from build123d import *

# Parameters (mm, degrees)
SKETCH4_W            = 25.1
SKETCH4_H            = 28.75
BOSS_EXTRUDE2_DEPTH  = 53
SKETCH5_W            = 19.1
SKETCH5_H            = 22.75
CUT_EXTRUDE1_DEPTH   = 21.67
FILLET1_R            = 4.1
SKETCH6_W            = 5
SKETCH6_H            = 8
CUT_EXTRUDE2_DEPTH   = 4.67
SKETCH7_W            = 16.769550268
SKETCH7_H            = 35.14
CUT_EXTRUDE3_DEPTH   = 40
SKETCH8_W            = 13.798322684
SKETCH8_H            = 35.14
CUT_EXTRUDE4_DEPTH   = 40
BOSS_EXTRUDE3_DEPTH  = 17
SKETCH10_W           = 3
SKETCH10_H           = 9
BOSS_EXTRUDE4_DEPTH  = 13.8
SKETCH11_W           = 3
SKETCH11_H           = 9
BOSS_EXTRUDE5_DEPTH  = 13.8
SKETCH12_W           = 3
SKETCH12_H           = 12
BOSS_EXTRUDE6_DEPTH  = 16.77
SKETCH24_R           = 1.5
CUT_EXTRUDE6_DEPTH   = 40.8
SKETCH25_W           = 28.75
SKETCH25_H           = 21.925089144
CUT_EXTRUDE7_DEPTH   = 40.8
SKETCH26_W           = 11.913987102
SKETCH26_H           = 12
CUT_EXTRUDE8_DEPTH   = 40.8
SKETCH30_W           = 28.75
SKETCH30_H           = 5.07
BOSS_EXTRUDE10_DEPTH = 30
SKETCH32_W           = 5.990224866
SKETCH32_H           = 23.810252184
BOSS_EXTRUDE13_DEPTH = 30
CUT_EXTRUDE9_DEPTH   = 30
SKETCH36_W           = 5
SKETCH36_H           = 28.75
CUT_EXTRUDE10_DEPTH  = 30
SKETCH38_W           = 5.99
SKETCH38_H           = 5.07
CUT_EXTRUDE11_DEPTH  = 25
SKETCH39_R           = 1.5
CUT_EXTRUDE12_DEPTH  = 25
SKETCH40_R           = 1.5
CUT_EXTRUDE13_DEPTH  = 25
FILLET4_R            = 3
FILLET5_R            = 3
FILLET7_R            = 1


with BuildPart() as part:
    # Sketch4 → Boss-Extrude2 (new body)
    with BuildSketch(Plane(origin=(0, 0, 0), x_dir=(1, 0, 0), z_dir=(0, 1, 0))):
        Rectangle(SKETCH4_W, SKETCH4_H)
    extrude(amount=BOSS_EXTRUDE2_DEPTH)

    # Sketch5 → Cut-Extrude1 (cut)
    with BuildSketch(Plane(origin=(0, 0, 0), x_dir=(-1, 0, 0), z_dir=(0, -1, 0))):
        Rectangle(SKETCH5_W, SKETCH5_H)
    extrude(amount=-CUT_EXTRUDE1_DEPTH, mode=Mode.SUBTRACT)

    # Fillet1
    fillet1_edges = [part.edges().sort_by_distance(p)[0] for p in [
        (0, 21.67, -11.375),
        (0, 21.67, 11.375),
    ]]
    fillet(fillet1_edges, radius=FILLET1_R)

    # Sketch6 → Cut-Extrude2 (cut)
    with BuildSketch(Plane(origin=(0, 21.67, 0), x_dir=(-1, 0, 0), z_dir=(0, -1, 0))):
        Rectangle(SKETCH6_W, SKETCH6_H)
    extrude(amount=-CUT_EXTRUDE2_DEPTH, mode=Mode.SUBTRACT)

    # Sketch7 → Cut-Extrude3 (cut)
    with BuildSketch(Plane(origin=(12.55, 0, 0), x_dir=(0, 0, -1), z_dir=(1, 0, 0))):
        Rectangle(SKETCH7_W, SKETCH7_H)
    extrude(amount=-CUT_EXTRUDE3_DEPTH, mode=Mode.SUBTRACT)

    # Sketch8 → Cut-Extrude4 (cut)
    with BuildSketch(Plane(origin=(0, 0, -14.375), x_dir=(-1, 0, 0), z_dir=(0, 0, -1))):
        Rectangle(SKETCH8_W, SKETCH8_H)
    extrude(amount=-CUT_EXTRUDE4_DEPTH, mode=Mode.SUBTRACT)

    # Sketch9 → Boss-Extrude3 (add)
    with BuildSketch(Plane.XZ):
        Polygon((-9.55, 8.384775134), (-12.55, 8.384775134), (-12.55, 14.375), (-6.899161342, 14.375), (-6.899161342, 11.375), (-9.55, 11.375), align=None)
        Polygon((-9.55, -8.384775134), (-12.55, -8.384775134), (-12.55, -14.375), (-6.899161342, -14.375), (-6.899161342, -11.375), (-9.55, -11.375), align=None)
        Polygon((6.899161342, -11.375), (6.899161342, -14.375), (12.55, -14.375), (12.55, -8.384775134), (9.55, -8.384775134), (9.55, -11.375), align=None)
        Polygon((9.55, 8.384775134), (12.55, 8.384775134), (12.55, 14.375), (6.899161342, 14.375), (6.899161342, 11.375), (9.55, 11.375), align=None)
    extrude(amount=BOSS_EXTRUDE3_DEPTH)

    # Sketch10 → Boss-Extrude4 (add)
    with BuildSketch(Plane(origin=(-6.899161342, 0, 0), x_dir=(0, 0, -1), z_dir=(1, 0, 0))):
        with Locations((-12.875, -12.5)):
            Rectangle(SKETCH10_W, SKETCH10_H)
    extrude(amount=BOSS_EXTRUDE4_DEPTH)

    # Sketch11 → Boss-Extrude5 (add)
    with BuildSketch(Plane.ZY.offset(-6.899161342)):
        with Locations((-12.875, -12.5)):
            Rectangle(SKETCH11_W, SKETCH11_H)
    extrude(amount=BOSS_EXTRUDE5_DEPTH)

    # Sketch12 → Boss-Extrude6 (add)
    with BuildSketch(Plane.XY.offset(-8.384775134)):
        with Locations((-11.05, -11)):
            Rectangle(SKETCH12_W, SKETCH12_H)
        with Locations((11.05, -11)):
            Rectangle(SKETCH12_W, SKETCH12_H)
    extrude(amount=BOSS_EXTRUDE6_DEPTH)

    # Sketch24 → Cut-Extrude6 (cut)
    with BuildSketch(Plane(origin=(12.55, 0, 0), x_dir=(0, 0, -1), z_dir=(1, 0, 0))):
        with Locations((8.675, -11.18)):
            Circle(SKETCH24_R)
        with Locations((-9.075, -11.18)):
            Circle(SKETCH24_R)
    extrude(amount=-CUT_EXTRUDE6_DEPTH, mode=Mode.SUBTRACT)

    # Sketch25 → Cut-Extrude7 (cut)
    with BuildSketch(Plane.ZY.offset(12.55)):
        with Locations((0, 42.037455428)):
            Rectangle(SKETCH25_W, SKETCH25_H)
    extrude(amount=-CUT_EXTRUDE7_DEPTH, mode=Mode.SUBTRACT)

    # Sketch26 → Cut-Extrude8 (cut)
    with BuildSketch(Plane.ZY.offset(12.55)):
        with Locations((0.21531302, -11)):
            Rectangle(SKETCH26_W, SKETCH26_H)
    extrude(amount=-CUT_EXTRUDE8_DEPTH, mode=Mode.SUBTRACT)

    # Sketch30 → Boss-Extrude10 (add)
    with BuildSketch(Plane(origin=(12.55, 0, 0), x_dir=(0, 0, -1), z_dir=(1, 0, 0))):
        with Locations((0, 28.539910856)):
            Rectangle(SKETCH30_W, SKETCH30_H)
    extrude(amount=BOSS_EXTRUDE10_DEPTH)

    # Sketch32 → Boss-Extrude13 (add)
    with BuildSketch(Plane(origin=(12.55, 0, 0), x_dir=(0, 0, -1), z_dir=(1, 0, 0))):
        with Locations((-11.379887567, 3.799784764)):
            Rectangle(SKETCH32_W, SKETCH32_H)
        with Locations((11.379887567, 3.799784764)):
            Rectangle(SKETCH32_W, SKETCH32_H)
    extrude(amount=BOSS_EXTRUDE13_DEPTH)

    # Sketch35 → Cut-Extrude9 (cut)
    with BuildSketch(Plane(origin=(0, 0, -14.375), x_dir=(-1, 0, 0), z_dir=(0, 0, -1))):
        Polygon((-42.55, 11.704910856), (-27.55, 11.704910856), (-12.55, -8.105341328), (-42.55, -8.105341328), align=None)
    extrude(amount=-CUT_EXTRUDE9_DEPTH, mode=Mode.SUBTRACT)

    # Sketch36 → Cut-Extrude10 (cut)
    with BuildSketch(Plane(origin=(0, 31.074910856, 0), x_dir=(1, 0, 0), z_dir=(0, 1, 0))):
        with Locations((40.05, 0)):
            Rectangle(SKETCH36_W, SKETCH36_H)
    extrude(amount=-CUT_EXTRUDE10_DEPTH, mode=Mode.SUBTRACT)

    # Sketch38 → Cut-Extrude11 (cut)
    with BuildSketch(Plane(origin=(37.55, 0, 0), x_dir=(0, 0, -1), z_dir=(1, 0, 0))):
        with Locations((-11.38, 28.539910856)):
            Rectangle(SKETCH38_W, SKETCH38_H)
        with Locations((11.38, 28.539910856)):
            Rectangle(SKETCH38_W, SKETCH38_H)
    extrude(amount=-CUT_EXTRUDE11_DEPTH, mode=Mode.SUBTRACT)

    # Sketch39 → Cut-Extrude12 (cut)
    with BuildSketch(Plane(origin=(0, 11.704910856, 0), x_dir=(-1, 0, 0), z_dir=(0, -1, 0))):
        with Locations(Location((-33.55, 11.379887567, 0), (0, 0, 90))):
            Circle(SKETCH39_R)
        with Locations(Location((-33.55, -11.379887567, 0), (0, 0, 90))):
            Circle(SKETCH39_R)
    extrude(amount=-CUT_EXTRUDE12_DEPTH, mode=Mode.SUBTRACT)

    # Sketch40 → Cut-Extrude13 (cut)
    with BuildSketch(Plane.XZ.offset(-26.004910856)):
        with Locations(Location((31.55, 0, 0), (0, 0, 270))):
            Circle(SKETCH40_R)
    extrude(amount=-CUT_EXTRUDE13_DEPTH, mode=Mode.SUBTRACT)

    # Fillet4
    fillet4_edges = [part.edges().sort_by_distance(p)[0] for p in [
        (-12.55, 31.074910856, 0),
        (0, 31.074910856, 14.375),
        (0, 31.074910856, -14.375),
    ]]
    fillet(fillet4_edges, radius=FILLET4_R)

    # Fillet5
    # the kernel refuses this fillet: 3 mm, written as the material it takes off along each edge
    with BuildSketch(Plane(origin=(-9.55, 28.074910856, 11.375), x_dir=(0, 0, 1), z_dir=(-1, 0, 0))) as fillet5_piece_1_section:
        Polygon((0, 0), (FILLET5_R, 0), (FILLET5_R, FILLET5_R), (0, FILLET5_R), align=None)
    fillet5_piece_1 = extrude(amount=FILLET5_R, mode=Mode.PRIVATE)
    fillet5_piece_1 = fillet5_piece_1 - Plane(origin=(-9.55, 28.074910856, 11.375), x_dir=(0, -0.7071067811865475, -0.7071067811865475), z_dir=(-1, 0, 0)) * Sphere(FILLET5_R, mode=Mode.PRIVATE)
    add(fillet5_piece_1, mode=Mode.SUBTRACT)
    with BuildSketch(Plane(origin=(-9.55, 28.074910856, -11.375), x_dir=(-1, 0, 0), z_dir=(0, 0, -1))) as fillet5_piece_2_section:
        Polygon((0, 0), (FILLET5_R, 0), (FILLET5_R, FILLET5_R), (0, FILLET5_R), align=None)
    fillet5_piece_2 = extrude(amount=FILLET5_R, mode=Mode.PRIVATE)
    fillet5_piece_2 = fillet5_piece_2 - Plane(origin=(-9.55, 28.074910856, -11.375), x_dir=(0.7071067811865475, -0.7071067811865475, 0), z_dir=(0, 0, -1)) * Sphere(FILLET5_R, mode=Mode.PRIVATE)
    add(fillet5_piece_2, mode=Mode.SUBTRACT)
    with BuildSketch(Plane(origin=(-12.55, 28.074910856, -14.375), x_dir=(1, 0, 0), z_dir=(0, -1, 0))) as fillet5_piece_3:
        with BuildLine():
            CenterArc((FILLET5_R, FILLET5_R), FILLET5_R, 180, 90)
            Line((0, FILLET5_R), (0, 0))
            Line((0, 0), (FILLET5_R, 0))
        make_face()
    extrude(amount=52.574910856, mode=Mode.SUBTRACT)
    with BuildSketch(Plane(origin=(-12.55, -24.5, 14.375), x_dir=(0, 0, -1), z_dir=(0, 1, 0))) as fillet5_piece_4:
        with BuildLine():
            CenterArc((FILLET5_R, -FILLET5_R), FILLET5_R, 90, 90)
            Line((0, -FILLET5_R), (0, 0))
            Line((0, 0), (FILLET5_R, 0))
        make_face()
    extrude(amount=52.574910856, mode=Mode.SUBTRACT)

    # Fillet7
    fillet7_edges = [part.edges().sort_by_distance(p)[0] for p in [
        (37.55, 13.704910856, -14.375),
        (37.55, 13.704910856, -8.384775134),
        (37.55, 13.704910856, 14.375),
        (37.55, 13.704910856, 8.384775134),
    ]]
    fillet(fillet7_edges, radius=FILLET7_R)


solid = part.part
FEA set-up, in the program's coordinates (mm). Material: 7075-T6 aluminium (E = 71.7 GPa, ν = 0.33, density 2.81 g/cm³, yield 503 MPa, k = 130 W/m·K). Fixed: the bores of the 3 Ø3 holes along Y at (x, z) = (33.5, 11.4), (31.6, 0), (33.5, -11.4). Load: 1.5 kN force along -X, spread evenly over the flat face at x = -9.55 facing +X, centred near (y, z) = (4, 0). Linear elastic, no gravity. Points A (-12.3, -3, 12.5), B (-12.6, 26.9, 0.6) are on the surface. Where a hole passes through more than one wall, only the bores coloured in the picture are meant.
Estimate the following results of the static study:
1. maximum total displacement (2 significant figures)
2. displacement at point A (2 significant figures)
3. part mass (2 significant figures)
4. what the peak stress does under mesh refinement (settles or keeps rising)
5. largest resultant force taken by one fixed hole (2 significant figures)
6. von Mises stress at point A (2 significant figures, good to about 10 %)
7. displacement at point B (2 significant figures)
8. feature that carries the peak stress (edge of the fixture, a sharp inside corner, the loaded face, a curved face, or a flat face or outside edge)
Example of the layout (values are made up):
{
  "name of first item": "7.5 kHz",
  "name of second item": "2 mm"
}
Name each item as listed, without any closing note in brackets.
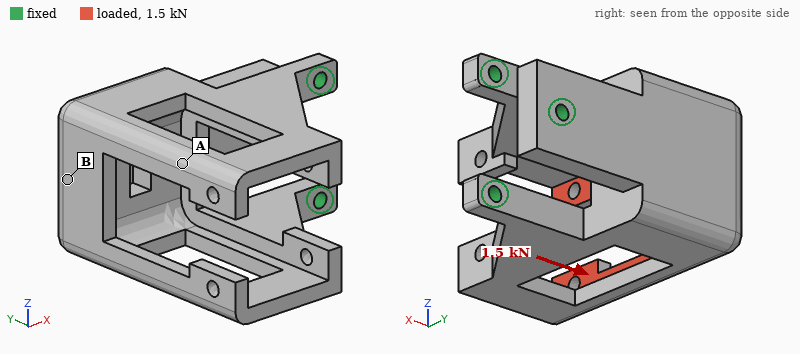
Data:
{
  "maximum total displacement": "0.21 mm",
  "displacement at point A": "0.13 mm",
  "part mass": "48 g",
  "what the peak stress does under mesh refinement": "keeps rising",
  "largest resultant force taken by one fixed hole": "1.1 kN",
  "von Mises stress at point A": "41 MPa",
  "displacement at point B": "0.083 mm",
  "feature that carries the peak stress": "edge of the fixture"
}
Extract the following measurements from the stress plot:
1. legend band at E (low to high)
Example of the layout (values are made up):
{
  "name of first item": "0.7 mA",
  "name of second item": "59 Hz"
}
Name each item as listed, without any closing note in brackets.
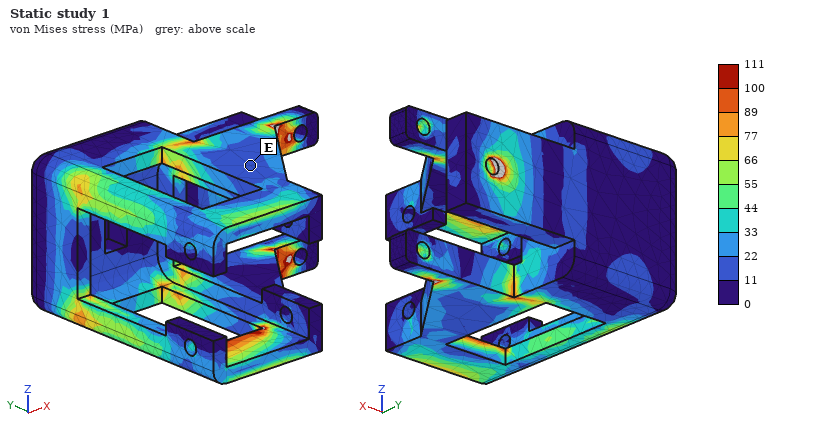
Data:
{
  "legend band at E": "11 to 22 MPa"
}
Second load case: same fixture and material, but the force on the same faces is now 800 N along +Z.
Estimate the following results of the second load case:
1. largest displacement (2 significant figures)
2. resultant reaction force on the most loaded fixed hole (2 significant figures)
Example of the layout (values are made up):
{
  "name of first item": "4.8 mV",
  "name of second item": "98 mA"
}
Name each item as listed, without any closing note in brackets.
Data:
{
  "largest displacement": "0.87 mm",
  "resultant reaction force on the most loaded fixed hole": "570 N"
}
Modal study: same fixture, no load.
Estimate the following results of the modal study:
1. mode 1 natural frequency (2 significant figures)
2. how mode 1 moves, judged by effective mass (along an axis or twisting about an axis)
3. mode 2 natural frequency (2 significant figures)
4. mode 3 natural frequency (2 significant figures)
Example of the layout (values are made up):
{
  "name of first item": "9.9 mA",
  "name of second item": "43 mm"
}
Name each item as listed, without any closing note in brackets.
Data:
{
  "mode 1 natural frequency": "1600 Hz",
  "how mode 1 moves, judged by effective mass": "along Z",
  "mode 2 natural frequency": "2600 Hz",
  "mode 3 natural frequency": "2700 Hz"
}
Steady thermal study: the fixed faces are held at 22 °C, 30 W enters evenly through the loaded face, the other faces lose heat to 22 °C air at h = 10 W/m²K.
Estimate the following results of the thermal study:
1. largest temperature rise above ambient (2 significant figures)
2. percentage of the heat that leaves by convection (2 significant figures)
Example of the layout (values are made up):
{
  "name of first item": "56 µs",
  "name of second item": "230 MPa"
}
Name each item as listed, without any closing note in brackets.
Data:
{
  "largest temperature rise above ambient": "72 K",
  "percentage of the heat that leaves by convection": "10 %"
}
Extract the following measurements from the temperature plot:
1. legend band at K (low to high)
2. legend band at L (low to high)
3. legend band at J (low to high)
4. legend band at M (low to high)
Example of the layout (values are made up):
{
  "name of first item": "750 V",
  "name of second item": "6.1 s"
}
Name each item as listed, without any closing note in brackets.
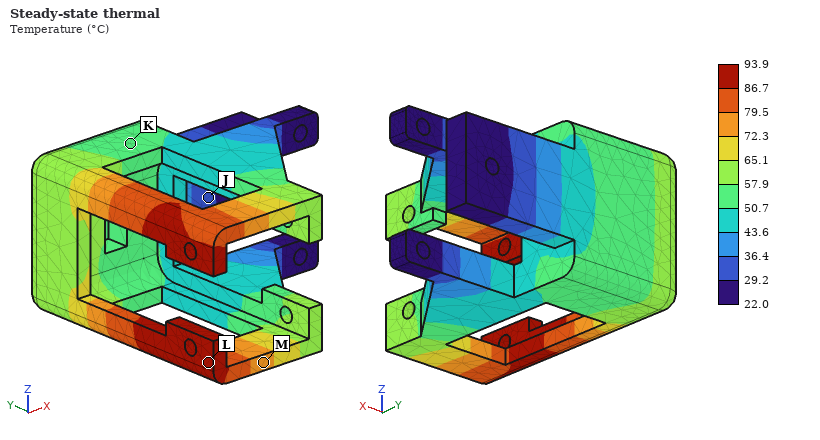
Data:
{
  "legend band at K": "50.7 to 57.9 °C",
  "legend band at L": "86.7 to 93.9 °C",
  "legend band at J": "29.2 to 36.4 °C",
  "legend band at M": "72.3 to 79.5 °C"
}
